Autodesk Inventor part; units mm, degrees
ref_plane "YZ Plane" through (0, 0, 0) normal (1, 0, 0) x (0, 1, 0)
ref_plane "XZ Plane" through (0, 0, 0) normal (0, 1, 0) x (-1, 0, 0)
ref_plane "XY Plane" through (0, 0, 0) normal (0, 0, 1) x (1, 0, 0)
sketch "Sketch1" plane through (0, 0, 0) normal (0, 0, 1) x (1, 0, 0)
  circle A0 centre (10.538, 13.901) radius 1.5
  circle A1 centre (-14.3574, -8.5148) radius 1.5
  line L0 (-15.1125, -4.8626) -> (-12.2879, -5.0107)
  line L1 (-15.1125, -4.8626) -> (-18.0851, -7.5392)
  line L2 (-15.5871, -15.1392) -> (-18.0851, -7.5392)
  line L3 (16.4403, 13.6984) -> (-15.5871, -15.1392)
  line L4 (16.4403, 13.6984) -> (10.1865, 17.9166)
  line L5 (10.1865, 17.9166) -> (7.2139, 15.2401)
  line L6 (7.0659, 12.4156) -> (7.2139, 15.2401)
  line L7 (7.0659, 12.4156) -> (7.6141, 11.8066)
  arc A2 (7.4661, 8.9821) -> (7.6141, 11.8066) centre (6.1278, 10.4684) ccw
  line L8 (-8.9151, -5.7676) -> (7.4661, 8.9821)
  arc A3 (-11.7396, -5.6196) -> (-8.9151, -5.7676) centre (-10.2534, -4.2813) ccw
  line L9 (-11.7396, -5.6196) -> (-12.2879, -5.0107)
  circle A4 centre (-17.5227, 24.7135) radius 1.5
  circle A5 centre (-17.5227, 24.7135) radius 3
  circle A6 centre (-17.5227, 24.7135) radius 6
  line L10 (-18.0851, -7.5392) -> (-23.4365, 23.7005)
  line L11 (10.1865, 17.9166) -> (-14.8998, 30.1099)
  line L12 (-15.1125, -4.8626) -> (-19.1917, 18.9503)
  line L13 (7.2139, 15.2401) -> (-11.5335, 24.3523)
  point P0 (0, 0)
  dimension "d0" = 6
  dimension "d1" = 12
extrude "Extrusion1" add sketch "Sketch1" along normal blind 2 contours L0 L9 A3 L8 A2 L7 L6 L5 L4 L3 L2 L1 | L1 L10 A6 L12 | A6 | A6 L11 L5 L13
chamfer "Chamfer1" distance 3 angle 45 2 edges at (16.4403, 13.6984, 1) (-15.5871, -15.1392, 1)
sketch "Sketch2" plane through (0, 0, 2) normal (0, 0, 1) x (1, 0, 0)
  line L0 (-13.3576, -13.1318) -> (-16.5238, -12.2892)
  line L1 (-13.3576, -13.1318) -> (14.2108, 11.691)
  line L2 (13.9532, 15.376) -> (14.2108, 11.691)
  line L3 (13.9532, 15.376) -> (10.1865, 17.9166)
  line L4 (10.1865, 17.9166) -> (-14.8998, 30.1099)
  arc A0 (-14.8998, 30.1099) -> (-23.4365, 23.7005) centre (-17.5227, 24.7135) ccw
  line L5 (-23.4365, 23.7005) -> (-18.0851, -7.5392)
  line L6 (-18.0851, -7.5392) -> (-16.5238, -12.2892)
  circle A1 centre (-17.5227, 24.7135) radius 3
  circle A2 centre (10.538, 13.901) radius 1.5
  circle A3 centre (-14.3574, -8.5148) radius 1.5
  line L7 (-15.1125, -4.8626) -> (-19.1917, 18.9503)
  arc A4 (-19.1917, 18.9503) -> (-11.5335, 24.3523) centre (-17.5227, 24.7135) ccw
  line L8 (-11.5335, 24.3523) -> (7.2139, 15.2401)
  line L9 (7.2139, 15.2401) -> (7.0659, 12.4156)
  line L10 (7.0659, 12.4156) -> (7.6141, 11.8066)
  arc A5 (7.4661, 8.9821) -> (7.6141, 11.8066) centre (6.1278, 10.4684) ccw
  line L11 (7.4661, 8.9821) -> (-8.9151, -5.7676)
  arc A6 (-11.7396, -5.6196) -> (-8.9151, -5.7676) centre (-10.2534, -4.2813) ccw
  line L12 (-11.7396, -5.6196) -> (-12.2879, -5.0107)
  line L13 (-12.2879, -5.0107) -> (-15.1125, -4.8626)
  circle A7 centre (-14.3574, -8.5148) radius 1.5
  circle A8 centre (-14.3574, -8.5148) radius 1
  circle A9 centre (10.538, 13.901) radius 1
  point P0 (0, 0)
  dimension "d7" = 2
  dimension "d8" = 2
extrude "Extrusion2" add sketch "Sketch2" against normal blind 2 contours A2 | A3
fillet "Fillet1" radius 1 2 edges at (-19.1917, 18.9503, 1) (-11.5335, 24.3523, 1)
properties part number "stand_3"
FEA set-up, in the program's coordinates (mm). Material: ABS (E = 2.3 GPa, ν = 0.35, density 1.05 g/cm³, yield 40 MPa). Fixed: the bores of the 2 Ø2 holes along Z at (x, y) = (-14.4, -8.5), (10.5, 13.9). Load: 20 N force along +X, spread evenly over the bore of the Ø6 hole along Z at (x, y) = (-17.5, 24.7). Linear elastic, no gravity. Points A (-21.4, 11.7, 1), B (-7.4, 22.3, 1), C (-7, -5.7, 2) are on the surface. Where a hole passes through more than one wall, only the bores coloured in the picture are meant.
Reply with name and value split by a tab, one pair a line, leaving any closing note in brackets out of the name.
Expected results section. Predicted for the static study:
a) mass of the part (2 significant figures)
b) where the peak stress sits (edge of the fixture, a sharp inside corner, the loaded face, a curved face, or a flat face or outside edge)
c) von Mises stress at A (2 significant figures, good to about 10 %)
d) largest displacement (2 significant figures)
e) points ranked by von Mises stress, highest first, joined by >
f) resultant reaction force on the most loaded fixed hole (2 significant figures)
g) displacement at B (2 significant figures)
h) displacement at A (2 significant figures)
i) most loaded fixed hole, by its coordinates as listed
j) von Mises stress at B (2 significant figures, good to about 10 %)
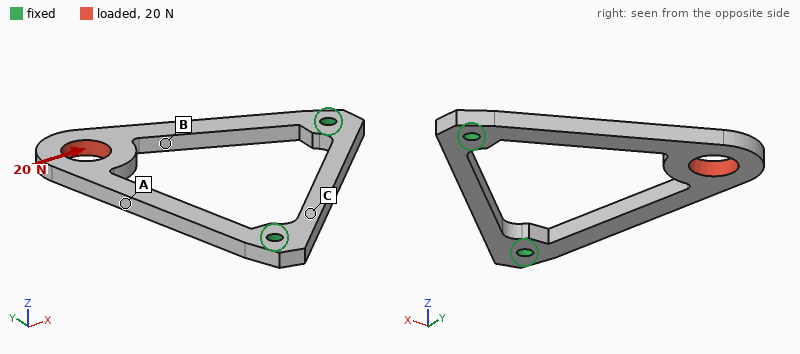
mass of the part	0.87 g
where the peak stress sits	a curved face
von Mises stress at A	3.5 MPa
largest displacement	0.20 mm
points ranked by von Mises stress, highest first, joined by >	B > A > C
resultant reaction force on the most loaded fixed hole	20 N
displacement at B	0.16 mm
displacement at A	0.17 mm
most loaded fixed hole, by its coordinates as listed	(10.5, 13.9)
von Mises stress at B	9.0 MPa
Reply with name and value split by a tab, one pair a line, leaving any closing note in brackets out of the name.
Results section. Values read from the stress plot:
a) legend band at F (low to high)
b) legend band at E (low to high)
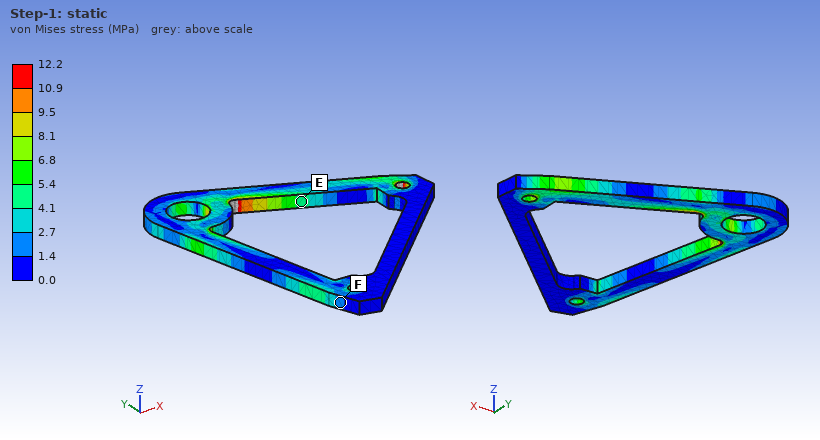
legend band at F	1.4 to 2.7 MPa
legend band at E	4.1 to 5.4 MPa
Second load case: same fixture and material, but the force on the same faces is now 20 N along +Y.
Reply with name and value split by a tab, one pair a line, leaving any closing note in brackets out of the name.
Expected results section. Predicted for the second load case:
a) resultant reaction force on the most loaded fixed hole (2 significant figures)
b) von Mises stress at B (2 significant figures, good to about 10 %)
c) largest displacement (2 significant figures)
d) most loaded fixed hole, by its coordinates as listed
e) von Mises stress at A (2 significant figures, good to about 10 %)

resultant reaction force on the most loaded fixed hole	18 N
von Mises stress at B	4.6 MPa
largest displacement	0.15 mm
most loaded fixed hole, by its coordinates as listed	(-14.4, -8.5)
von Mises stress at A	0.88 MPa
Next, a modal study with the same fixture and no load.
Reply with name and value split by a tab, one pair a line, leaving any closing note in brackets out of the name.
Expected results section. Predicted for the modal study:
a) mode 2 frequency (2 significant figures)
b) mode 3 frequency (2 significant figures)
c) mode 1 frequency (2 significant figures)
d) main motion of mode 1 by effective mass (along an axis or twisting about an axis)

mode 2 frequency	1600 Hz
mode 3 frequency	2300 Hz
mode 1 frequency	400 Hz
main motion of mode 1 by effective mass	along Z
